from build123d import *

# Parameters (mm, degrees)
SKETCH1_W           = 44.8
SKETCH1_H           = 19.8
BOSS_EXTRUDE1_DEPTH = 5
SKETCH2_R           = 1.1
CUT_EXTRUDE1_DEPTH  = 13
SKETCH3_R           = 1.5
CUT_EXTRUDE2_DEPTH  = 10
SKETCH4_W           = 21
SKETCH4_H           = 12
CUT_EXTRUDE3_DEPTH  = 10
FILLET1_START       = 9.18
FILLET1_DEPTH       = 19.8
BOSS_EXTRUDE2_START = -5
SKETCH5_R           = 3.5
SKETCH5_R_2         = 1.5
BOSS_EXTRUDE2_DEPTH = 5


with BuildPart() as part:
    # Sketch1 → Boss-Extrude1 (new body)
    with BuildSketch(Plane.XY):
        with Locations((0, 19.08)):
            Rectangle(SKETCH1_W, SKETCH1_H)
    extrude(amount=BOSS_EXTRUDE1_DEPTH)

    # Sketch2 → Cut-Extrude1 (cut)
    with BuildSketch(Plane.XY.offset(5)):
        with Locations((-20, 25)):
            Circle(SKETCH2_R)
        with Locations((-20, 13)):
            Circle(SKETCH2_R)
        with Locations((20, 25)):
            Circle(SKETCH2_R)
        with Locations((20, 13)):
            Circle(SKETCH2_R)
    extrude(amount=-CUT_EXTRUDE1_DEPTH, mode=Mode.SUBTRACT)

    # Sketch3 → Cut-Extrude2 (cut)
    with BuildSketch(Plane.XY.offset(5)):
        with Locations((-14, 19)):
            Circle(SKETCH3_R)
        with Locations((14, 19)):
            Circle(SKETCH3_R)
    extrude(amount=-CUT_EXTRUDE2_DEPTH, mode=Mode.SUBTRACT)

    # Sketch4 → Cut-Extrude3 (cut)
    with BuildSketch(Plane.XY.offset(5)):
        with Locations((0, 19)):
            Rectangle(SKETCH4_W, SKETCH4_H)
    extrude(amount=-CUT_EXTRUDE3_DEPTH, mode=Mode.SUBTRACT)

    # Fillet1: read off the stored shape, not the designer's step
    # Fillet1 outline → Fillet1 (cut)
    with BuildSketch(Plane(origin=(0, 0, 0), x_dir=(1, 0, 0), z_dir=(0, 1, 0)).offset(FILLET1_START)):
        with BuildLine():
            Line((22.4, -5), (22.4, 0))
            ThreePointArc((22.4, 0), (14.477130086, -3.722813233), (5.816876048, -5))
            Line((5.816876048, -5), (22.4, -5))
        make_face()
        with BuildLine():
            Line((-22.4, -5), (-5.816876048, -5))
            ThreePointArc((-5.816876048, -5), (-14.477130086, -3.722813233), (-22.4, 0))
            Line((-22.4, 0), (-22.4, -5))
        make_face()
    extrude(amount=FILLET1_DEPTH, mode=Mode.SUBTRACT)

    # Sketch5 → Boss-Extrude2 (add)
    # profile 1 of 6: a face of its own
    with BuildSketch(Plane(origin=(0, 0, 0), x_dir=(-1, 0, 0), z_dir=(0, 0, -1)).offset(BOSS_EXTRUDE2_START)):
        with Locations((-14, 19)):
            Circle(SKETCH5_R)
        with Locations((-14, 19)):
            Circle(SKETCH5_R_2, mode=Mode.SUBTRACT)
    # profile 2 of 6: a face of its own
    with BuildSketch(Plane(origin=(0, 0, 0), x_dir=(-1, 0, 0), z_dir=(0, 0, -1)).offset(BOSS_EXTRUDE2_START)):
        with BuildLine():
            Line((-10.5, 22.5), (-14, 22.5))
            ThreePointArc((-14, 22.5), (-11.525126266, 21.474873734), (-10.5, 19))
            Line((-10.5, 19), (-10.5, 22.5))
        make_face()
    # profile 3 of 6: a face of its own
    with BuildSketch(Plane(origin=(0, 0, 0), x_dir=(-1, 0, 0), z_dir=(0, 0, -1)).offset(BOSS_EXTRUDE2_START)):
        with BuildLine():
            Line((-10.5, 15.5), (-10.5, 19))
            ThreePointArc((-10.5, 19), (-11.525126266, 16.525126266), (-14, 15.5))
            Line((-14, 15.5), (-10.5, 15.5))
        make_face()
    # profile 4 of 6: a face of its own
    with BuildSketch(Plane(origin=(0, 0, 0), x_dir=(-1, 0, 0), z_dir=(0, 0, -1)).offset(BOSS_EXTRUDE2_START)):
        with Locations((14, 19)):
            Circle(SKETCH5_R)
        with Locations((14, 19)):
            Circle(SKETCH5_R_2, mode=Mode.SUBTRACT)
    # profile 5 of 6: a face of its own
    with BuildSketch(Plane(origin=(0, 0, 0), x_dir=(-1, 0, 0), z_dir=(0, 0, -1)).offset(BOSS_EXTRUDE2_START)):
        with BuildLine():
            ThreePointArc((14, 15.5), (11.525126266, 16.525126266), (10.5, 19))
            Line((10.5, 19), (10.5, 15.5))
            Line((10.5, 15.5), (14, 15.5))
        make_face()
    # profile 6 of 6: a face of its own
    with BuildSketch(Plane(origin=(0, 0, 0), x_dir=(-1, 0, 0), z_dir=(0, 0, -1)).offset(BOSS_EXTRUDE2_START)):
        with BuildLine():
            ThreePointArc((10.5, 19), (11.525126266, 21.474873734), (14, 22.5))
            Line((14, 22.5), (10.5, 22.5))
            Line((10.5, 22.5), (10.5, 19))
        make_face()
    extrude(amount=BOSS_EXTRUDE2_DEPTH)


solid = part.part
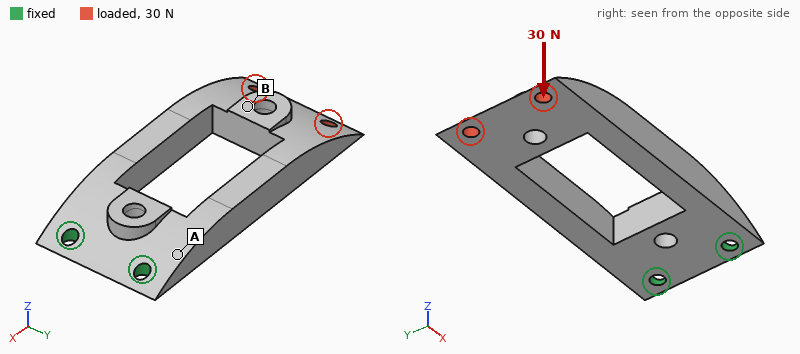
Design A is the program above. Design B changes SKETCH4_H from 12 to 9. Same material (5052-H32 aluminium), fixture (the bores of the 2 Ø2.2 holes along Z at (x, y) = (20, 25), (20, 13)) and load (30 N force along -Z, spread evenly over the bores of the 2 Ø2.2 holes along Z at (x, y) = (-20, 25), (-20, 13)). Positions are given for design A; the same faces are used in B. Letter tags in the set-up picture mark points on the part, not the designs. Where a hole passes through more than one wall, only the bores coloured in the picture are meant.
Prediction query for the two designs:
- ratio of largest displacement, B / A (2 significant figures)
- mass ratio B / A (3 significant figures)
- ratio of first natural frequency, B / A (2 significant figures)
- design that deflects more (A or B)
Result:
0.91
1.15
0.98
A
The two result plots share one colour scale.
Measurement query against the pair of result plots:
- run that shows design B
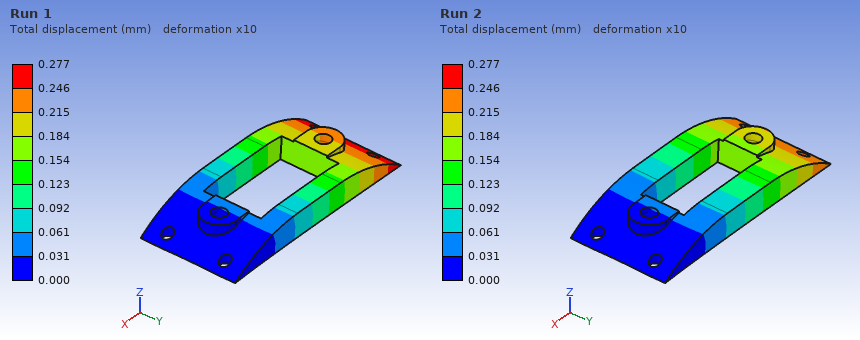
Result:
Run 2
